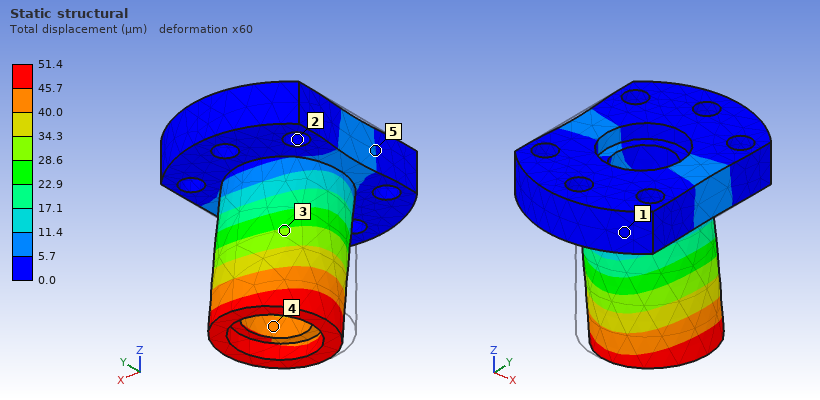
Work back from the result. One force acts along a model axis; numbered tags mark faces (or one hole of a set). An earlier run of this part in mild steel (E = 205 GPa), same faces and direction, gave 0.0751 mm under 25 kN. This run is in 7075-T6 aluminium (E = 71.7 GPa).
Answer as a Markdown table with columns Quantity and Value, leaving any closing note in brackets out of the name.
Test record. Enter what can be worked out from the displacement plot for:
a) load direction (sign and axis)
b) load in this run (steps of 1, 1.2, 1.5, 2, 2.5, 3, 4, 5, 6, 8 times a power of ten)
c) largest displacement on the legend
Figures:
| Quantity | Value |
|---|---|
| load direction | +X |
| load in this run | 6 kN |
| largest displacement on the legend | 51.4 µm |
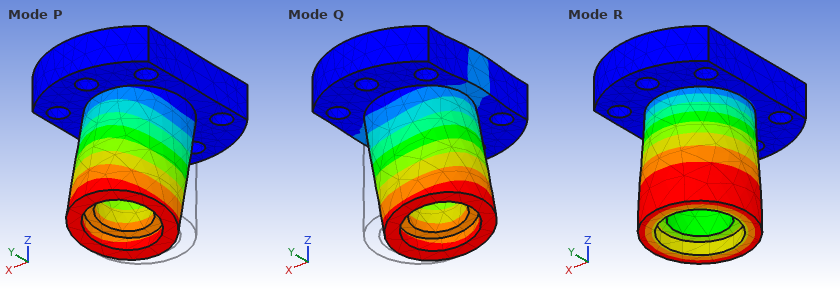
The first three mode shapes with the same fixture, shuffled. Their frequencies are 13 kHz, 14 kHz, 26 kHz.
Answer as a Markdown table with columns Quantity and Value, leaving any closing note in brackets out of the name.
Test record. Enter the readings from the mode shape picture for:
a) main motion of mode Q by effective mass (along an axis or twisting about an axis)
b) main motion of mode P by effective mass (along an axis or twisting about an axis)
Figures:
| Quantity | Value |
|---|---|
| main motion of mode Q by effective mass | along X |
| main motion of mode P by effective mass | along Y |
